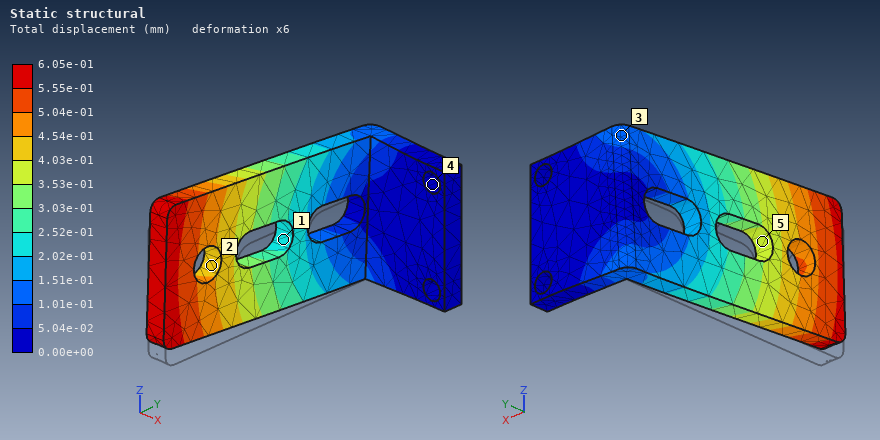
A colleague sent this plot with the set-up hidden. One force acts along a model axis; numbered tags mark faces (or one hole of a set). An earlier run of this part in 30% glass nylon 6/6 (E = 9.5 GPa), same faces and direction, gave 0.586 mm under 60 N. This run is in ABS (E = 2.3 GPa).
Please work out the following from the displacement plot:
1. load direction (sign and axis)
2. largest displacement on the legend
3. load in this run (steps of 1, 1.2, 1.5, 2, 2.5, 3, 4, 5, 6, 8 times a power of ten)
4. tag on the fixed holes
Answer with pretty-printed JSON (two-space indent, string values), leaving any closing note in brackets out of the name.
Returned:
{
  "load direction": "+Z",
  "largest displacement on the legend": "6.05e-01 mm",
  "load in this run": "15 N",
  "tag on the fixed holes": "4"
}
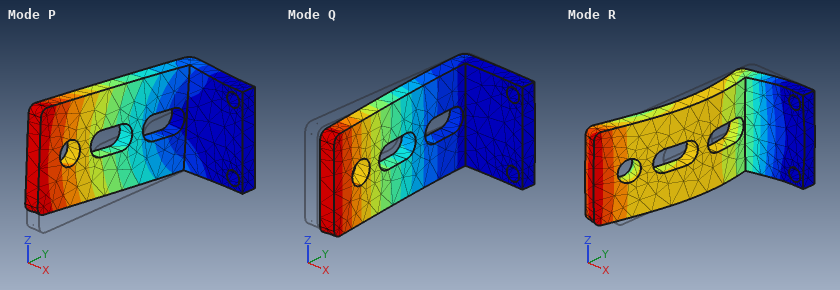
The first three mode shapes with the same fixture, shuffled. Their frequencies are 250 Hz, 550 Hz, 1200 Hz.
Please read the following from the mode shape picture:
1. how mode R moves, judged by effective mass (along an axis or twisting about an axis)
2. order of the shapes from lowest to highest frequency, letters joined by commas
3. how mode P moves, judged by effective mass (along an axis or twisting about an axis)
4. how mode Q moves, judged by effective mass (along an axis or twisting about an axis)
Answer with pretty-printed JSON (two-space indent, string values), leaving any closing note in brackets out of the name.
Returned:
{
  "how mode R moves, judged by effective mass": "along Y",
  "order of the shapes from lowest to highest frequency, letters joined by commas": "Q, P, R",
  "how mode P moves, judged by effective mass": "along Z",
  "how mode Q moves, judged by effective mass": "along X"
}
